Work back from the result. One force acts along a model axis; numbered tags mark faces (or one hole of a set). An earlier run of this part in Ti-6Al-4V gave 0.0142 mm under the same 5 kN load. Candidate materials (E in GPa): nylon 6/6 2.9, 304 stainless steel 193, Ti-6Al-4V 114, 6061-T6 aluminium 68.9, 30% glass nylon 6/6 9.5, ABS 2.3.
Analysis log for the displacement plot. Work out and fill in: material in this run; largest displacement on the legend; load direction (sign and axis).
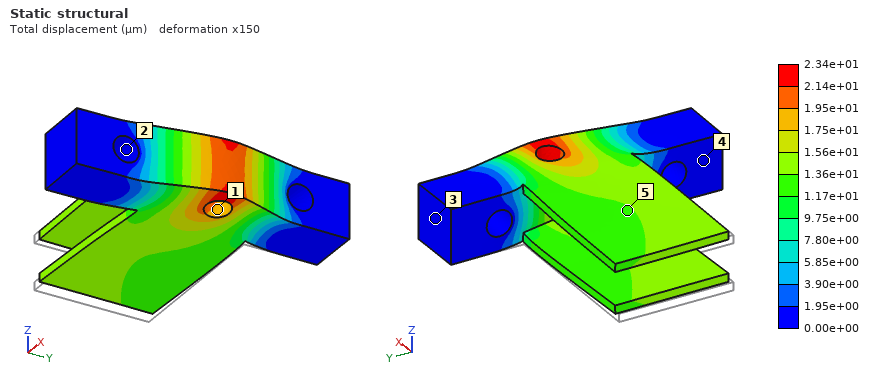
6061-T6 aluminium
2.34e+01 µm
+X
